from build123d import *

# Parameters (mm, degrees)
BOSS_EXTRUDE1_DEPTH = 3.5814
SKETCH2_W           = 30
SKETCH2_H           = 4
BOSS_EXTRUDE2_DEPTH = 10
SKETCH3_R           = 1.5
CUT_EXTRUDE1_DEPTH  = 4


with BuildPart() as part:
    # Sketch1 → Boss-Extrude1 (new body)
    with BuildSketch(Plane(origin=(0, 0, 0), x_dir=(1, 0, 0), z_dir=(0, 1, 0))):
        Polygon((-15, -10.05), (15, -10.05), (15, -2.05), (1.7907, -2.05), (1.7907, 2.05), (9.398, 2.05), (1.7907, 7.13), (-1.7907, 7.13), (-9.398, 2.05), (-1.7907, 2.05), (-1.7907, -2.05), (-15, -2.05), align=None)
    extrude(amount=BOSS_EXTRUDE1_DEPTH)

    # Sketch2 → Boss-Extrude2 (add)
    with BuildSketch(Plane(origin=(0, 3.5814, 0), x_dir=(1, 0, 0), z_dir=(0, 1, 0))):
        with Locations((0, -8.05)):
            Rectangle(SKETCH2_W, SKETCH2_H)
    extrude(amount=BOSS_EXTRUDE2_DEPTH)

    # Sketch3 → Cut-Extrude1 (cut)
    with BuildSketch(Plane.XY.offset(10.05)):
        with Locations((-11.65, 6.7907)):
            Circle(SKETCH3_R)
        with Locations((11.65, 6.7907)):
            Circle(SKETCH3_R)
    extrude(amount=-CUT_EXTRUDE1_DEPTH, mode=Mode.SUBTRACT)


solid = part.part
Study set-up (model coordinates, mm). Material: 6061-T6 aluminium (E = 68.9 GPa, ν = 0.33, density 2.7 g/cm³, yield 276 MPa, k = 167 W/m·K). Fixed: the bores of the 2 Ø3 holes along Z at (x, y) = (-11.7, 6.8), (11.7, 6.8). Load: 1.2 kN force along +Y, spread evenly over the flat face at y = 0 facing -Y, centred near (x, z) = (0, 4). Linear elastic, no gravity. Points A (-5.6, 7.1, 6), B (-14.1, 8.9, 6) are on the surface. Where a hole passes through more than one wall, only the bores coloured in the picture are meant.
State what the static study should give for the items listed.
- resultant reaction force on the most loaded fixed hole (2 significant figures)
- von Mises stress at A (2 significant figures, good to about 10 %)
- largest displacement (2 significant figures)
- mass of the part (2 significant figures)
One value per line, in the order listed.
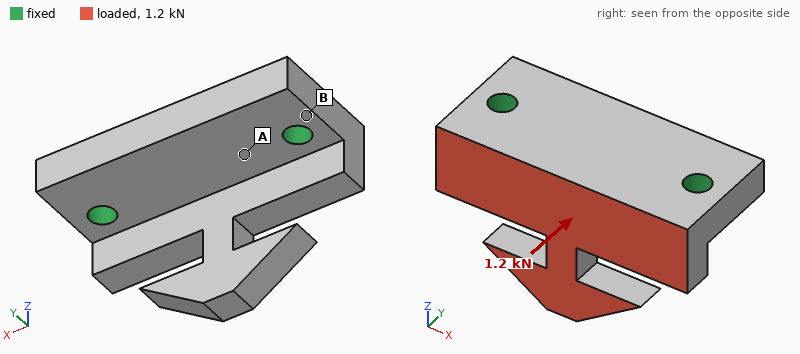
600 N
43 MPa
0.16 mm
6.1 g
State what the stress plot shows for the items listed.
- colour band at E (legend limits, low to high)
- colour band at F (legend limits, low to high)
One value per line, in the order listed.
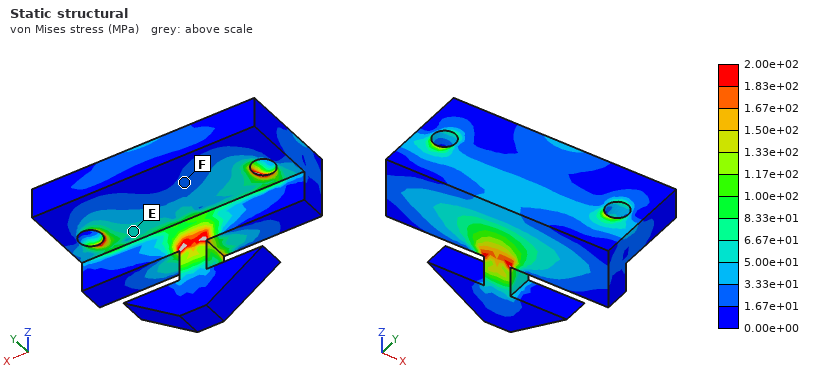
5.00e+01 to 6.67e+01 MPa
1.67e+01 to 3.33e+01 MPa
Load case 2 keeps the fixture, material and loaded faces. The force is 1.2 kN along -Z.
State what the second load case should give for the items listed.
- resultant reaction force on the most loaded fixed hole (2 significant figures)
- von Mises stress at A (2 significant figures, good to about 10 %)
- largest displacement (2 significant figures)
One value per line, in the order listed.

620 N
39 MPa
98 µm
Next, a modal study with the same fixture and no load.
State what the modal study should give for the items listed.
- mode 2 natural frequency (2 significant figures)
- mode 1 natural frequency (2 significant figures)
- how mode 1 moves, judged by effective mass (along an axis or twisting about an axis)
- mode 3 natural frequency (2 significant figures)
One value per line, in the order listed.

13 kHz
10000 Hz
along Y
17 kHz
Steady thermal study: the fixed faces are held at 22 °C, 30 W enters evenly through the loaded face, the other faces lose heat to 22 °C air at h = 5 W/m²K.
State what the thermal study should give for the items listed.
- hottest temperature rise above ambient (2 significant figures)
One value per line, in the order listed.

39 K
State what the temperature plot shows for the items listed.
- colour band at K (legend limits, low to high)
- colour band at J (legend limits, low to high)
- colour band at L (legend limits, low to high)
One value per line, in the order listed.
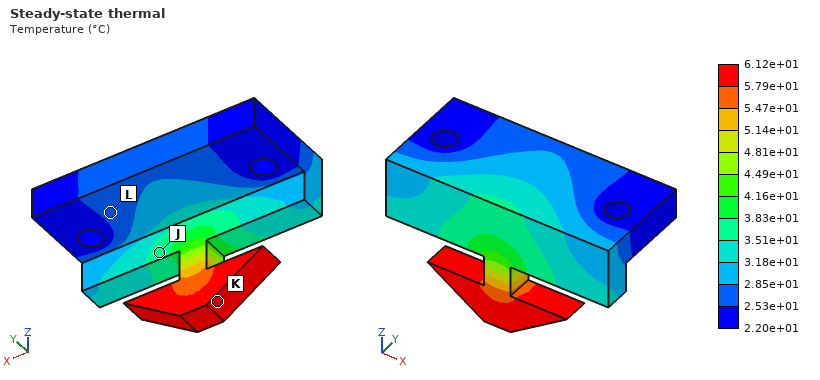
5.79e+01 to 6.12e+01 °C
3.51e+01 to 3.83e+01 °C
2.53e+01 to 2.85e+01 °C
